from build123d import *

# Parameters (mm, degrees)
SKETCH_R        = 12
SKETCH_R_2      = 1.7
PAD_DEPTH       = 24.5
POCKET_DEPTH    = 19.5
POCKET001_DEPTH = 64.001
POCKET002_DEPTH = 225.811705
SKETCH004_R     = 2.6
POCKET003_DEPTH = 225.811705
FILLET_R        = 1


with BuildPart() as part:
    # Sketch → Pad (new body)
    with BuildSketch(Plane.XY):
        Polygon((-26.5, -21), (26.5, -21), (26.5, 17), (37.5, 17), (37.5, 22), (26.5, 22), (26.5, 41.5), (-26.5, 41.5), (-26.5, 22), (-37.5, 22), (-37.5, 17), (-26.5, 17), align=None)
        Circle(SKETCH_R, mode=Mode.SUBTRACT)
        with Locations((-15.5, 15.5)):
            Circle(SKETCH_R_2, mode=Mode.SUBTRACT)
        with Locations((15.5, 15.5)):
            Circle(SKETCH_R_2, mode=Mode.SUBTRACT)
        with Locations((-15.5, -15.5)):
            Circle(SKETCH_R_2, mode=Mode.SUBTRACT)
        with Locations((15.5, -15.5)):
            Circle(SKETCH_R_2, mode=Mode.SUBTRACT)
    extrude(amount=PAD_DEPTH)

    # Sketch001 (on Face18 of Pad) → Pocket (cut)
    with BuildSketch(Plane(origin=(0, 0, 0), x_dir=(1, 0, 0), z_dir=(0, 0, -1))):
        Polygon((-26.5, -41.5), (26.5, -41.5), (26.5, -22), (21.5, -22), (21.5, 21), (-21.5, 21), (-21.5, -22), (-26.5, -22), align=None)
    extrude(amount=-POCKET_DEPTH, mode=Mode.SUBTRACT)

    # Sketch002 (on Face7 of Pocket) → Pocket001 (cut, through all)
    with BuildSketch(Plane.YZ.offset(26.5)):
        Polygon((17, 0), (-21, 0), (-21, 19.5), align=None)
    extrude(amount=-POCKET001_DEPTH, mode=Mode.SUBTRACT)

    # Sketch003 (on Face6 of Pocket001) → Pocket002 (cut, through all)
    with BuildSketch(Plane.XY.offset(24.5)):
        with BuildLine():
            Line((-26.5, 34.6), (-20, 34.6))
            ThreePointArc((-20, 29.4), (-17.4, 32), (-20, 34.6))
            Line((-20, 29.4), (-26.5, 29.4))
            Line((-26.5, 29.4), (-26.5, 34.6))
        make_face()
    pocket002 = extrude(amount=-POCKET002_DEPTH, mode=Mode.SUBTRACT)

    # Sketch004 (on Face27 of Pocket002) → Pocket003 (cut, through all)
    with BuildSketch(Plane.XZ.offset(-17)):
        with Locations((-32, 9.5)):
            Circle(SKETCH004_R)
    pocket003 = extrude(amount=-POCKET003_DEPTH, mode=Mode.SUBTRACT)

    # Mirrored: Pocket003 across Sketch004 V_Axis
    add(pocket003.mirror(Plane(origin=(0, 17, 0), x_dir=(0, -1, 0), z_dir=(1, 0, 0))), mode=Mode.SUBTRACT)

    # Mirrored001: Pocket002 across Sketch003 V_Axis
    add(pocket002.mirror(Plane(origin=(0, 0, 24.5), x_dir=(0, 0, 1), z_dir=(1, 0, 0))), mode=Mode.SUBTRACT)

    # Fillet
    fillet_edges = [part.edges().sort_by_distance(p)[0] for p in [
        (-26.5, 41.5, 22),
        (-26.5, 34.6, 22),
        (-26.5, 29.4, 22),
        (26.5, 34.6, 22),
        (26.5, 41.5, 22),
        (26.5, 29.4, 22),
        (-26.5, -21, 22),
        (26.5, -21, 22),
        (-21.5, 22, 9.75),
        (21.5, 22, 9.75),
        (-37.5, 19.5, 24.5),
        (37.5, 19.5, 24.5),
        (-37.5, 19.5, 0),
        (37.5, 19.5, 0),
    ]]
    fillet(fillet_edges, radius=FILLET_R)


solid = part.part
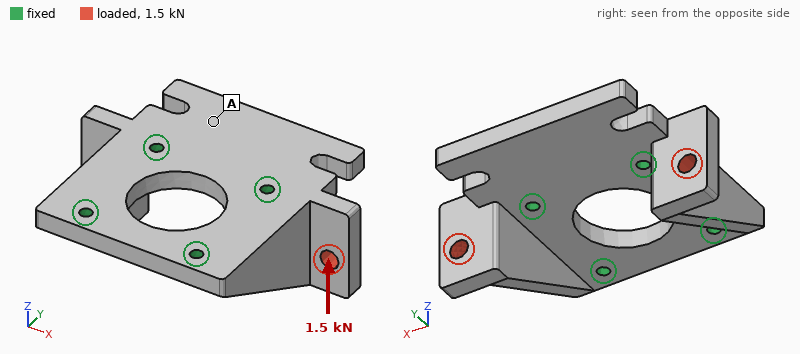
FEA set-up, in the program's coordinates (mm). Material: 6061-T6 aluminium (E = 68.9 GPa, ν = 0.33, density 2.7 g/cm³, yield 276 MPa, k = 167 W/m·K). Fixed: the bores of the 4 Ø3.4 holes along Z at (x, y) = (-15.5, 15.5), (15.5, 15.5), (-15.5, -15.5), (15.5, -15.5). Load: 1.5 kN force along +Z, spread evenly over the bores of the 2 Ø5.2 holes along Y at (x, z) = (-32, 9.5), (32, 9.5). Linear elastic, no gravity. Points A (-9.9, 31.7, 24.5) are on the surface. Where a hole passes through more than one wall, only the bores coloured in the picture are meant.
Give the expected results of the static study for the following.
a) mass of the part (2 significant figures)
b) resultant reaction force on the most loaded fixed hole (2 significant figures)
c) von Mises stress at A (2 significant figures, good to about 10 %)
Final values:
56 g
800 N
17 MPa
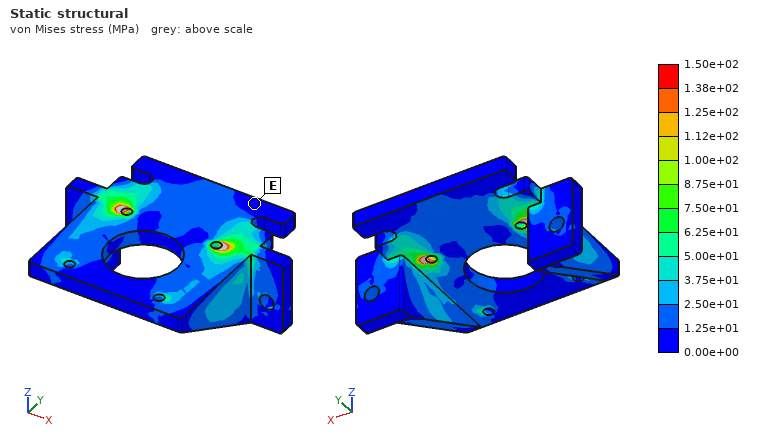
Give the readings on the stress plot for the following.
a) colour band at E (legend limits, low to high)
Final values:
0.00e+00 to 1.25e+01 MPa
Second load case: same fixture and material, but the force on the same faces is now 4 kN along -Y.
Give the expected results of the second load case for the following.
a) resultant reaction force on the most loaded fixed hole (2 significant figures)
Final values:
1.5 kN
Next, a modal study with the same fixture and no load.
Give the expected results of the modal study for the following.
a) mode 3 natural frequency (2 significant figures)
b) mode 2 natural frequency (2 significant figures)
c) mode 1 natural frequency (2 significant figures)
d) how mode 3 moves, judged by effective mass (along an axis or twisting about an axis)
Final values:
5500 Hz
5100 Hz
5000 Hz
along Z
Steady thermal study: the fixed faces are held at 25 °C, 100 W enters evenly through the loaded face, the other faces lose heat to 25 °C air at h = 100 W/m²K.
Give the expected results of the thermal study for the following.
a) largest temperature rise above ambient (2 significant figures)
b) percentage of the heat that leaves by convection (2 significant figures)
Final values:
66 K
17 %
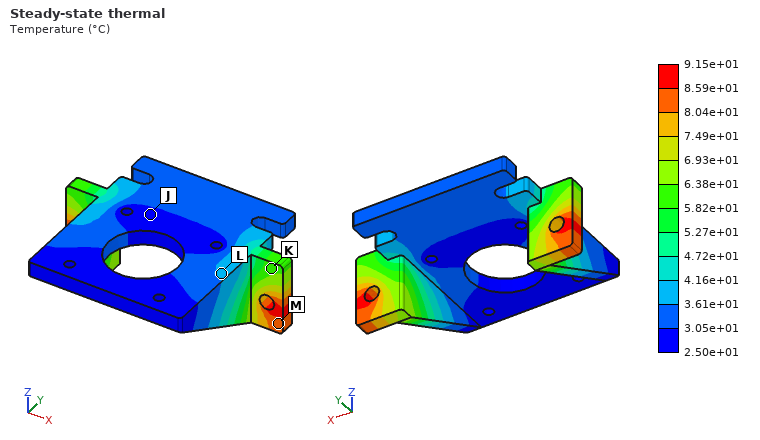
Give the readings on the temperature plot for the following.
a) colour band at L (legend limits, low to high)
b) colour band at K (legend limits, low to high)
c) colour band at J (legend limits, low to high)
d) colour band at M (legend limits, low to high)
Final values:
3.61e+01 to 4.16e+01 °C
5.82e+01 to 6.38e+01 °C
2.50e+01 to 3.05e+01 °C
8.04e+01 to 8.59e+01 °C
